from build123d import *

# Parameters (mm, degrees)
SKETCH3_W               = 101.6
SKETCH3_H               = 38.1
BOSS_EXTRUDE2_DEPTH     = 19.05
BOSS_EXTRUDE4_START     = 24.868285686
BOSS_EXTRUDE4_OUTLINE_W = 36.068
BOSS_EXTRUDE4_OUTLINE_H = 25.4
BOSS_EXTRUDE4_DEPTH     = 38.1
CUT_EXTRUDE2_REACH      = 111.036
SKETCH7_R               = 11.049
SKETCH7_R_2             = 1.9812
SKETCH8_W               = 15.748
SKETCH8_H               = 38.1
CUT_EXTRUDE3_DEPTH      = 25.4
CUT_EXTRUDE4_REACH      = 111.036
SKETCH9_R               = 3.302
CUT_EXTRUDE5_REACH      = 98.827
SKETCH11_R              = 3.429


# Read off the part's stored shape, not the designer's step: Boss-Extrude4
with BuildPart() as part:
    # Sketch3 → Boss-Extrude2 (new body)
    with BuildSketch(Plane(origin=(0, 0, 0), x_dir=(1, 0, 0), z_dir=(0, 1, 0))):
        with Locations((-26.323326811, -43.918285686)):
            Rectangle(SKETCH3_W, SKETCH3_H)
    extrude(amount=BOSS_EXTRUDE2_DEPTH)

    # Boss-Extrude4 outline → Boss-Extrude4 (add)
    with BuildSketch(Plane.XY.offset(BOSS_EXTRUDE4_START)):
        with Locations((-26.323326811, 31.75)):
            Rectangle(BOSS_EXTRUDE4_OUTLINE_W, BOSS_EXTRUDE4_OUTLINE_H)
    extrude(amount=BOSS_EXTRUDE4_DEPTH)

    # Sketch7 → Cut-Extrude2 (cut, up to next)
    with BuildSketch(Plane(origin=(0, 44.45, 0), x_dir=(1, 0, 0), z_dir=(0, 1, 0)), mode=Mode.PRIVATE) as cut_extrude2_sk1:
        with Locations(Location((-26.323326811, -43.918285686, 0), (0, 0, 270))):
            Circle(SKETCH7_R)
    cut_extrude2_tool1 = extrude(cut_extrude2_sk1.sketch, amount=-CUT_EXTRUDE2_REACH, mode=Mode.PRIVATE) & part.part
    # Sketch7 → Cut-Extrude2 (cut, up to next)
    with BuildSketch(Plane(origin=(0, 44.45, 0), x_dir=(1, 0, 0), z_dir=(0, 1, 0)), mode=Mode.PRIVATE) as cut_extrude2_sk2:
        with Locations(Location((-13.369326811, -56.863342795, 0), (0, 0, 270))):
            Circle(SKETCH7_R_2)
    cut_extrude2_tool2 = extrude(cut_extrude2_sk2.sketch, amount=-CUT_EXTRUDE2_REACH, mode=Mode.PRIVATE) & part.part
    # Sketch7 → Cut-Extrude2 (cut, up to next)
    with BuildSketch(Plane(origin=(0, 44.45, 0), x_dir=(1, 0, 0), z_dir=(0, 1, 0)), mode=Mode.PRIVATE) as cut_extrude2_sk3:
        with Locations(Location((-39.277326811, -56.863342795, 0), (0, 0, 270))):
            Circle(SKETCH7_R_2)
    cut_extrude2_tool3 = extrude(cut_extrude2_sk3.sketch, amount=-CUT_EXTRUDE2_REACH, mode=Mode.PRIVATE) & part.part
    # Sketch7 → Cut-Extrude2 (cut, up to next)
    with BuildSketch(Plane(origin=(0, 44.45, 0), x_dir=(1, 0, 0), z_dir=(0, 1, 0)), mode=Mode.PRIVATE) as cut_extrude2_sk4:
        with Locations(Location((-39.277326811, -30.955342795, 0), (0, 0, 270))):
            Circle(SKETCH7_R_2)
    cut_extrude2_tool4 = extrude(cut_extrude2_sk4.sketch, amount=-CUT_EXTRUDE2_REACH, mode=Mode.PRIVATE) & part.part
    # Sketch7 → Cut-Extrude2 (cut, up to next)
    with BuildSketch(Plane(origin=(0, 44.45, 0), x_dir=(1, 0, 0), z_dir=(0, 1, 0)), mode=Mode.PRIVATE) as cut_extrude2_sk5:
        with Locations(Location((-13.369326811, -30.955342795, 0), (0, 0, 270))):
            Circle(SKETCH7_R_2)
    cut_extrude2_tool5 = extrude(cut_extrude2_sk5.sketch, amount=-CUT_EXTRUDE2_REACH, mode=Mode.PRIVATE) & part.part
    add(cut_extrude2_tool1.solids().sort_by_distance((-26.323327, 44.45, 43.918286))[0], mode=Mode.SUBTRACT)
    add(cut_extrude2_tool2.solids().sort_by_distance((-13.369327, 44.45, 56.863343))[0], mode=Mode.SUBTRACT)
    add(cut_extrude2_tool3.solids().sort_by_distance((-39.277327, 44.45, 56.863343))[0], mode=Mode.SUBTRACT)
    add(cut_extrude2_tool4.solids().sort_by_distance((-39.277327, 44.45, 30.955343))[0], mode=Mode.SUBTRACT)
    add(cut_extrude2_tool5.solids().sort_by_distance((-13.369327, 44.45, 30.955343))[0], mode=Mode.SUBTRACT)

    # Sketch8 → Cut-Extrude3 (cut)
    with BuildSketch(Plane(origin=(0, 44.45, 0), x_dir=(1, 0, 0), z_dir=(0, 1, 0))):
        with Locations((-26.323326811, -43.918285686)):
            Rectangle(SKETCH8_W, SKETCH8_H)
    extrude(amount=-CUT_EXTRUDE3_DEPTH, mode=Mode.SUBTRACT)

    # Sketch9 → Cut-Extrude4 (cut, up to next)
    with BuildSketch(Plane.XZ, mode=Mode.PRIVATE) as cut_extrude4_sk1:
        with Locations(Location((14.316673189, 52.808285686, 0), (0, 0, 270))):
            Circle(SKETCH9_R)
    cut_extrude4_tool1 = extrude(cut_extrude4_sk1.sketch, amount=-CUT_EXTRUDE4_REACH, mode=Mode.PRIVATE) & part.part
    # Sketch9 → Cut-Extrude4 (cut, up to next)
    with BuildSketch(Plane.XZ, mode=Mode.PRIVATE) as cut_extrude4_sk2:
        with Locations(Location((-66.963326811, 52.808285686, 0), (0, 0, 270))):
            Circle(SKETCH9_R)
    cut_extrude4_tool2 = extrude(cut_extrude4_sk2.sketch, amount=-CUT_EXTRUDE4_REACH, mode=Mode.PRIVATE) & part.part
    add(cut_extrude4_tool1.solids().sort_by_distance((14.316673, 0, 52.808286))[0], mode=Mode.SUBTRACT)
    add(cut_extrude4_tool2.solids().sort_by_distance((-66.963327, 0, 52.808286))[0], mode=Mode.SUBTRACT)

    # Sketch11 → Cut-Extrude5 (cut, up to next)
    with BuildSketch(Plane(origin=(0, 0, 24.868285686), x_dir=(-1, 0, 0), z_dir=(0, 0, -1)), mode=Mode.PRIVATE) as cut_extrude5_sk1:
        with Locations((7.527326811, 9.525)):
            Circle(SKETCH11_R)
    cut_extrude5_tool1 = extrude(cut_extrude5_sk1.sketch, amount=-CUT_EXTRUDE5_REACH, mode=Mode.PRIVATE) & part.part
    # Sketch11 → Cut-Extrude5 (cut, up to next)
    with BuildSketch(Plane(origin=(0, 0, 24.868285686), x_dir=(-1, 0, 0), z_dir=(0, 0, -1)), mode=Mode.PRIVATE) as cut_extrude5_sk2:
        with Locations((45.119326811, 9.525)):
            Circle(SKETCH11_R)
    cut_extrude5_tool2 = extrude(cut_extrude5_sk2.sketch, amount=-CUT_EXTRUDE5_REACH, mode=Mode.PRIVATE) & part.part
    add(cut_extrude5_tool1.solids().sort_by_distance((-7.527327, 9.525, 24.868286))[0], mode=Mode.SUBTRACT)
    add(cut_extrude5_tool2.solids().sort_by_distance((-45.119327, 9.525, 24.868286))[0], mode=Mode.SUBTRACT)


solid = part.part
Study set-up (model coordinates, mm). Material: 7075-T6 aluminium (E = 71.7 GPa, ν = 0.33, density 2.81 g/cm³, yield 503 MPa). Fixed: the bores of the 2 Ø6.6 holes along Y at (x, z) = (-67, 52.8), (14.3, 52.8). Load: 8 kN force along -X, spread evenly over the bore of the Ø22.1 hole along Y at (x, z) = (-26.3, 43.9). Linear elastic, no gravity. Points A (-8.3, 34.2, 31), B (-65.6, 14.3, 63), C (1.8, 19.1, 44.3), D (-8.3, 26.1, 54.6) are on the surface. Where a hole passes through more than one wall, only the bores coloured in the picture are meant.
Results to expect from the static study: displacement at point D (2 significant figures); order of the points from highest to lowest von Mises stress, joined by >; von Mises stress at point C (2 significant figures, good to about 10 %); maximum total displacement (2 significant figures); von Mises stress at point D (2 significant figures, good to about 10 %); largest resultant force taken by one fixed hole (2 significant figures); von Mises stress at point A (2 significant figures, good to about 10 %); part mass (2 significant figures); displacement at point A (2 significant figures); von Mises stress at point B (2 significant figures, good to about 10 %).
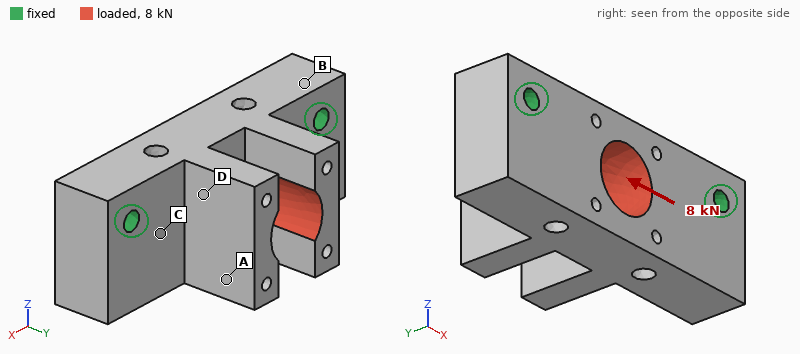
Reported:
13 µm
D > C > A > B
13 MPa
42 µm
17 MPa
4.2 kN
7.6 MPa
220 g
25 µm
3.7 MPa
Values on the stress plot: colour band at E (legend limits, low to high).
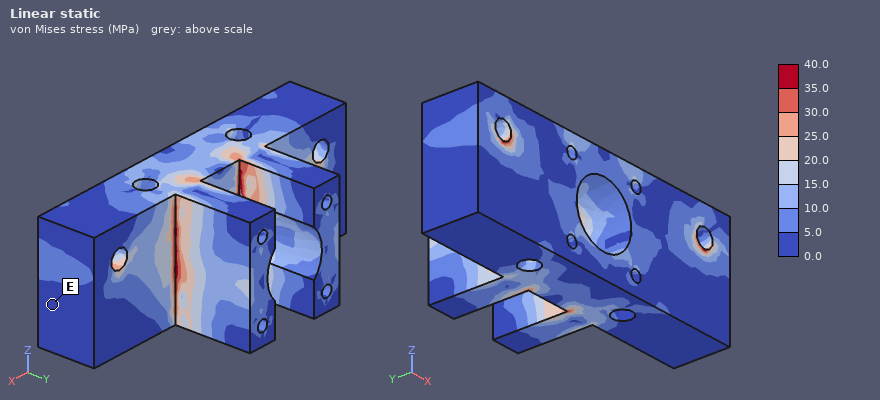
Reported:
0.0 to 5.0 MPa
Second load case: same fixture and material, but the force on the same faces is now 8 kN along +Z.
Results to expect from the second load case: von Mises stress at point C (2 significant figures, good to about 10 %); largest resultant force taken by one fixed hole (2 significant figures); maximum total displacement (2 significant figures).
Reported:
31 MPa
4.5 kN
56 µm
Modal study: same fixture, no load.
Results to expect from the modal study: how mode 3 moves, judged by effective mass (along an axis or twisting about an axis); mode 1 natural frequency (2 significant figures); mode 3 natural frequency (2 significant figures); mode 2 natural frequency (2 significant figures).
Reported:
along X
5800 Hz
8200 Hz
6800 Hz
